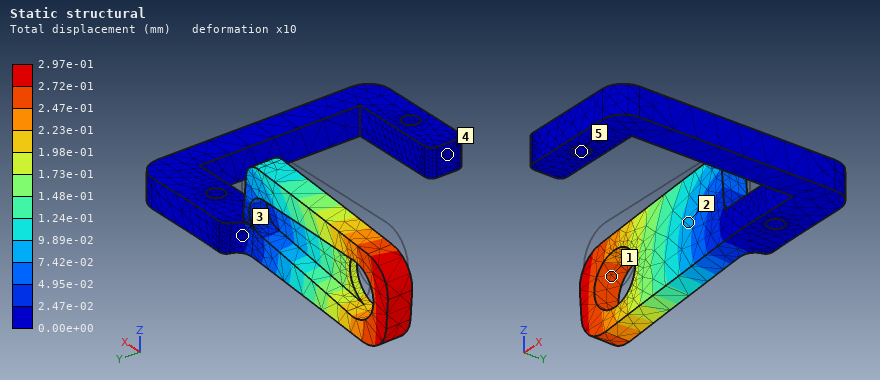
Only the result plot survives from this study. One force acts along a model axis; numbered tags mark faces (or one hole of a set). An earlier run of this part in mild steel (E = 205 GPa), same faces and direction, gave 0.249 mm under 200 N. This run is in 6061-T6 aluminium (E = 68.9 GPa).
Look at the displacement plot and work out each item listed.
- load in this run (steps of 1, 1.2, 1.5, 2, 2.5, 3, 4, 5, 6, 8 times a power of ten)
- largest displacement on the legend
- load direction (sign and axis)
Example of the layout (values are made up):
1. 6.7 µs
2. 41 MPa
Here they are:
1. 80 N
2. 2.97e-01 mm
3. -Z
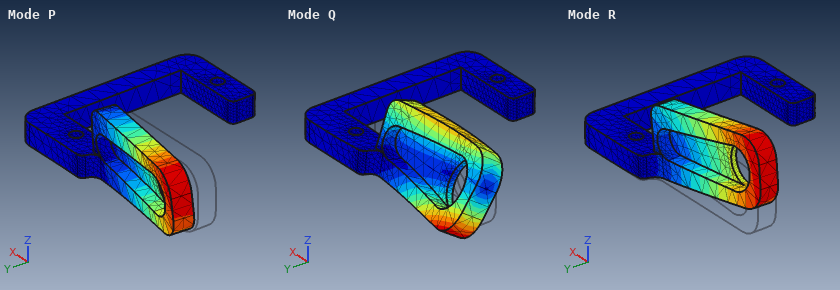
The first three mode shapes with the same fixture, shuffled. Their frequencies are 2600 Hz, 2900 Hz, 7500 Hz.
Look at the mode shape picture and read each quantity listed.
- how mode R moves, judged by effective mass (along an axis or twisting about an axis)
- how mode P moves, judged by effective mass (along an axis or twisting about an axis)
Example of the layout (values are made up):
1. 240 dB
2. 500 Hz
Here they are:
1. along Z
2. along Y
